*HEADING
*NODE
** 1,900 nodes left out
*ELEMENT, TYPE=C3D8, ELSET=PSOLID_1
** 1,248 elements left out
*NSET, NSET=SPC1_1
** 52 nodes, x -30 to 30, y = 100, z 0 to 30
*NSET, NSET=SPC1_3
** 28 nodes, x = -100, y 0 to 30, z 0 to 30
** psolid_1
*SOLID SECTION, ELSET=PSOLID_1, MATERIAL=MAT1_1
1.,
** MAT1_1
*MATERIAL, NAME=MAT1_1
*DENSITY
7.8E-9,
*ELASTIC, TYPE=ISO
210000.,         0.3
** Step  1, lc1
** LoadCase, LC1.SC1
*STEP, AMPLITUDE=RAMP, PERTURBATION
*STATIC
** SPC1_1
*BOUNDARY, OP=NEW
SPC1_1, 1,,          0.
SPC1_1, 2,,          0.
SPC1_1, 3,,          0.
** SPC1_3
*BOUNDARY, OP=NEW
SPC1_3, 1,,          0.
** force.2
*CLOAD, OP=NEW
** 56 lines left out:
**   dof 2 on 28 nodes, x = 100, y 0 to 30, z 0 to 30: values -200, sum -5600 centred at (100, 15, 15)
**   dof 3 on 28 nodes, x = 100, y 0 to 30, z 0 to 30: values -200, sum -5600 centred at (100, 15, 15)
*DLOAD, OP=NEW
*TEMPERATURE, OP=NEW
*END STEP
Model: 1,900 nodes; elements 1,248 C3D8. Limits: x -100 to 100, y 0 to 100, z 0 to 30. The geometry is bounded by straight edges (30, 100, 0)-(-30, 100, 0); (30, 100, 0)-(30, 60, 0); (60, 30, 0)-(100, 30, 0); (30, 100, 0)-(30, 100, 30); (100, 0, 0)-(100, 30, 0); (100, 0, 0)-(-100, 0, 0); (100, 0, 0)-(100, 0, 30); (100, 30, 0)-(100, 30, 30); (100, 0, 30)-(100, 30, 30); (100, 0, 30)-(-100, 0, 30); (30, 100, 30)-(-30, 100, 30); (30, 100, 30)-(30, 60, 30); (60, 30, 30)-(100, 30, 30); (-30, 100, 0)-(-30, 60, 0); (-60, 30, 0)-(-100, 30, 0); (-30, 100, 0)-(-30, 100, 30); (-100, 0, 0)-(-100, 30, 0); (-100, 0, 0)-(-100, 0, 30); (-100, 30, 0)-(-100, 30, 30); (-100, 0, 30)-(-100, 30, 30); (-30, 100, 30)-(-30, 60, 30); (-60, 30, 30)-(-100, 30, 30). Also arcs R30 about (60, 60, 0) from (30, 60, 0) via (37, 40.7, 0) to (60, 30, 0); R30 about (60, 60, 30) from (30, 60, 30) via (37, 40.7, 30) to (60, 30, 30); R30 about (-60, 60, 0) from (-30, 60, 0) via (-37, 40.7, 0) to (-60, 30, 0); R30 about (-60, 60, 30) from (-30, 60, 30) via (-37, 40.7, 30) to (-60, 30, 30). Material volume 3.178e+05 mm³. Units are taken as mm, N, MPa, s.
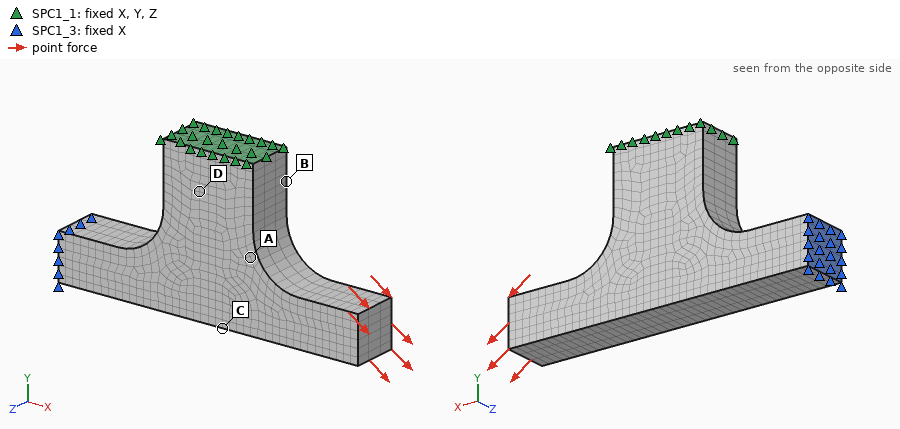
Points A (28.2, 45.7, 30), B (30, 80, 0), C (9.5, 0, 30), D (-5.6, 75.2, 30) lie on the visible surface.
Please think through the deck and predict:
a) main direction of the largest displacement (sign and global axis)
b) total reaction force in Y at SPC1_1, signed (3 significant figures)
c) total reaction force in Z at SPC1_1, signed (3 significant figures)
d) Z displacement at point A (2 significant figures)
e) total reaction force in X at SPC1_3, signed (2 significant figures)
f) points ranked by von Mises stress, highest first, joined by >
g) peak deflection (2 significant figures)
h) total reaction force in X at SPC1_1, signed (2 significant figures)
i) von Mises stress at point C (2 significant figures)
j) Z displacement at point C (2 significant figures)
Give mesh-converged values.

-Z
5600 N
5600 N
-0.042 mm
6100 N
A > D > B > C
0.23 mm
-6100 N
18 MPa
-0.053 mm
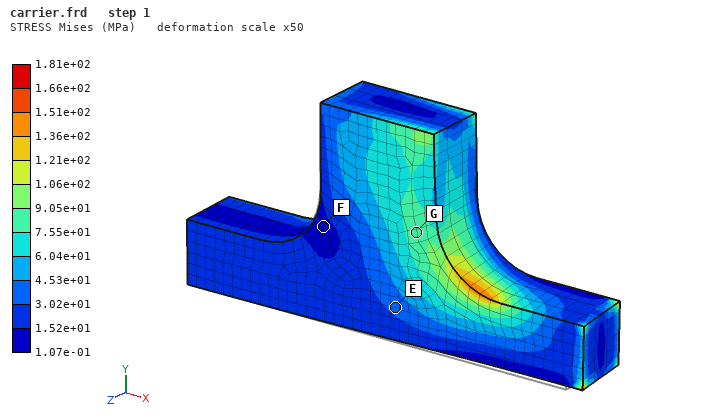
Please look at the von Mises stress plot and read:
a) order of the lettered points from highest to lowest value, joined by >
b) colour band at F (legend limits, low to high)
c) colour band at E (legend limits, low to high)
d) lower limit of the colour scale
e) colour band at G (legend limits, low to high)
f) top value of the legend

G > E > F
1.07e-01 to 1.52e+01 MPa
3.02e+01 to 4.53e+01 MPa
1.07e-01 MPa
7.55e+01 to 9.05e+01 MPa
1.81e+02 MPa
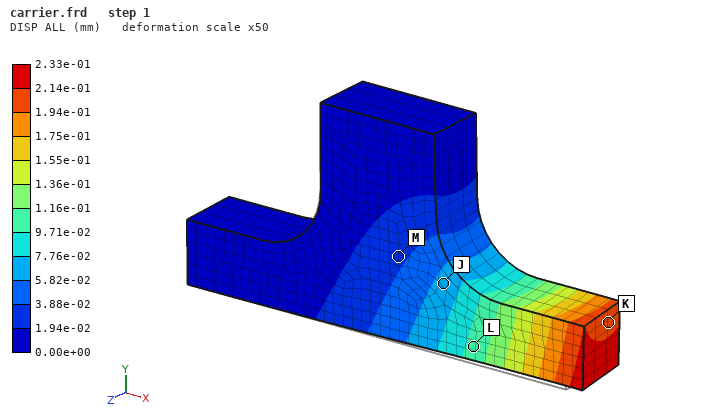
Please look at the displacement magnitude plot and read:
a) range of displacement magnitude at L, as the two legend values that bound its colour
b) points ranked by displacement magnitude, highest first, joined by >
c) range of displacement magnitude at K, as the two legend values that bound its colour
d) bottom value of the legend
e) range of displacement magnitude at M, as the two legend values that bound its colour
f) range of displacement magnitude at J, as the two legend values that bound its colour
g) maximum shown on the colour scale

9.71e-02 to 1.16e-01 mm
K > L > J > M
1.94e-01 to 2.14e-01 mm
0.00e+00 mm
1.94e-02 to 3.88e-02 mm
5.82e-02 to 7.76e-02 mm
2.33e-01 mm
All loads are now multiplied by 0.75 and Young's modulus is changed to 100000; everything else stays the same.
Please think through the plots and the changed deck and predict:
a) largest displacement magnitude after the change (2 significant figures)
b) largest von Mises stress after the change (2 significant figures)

0.37 mm
140 MPa
